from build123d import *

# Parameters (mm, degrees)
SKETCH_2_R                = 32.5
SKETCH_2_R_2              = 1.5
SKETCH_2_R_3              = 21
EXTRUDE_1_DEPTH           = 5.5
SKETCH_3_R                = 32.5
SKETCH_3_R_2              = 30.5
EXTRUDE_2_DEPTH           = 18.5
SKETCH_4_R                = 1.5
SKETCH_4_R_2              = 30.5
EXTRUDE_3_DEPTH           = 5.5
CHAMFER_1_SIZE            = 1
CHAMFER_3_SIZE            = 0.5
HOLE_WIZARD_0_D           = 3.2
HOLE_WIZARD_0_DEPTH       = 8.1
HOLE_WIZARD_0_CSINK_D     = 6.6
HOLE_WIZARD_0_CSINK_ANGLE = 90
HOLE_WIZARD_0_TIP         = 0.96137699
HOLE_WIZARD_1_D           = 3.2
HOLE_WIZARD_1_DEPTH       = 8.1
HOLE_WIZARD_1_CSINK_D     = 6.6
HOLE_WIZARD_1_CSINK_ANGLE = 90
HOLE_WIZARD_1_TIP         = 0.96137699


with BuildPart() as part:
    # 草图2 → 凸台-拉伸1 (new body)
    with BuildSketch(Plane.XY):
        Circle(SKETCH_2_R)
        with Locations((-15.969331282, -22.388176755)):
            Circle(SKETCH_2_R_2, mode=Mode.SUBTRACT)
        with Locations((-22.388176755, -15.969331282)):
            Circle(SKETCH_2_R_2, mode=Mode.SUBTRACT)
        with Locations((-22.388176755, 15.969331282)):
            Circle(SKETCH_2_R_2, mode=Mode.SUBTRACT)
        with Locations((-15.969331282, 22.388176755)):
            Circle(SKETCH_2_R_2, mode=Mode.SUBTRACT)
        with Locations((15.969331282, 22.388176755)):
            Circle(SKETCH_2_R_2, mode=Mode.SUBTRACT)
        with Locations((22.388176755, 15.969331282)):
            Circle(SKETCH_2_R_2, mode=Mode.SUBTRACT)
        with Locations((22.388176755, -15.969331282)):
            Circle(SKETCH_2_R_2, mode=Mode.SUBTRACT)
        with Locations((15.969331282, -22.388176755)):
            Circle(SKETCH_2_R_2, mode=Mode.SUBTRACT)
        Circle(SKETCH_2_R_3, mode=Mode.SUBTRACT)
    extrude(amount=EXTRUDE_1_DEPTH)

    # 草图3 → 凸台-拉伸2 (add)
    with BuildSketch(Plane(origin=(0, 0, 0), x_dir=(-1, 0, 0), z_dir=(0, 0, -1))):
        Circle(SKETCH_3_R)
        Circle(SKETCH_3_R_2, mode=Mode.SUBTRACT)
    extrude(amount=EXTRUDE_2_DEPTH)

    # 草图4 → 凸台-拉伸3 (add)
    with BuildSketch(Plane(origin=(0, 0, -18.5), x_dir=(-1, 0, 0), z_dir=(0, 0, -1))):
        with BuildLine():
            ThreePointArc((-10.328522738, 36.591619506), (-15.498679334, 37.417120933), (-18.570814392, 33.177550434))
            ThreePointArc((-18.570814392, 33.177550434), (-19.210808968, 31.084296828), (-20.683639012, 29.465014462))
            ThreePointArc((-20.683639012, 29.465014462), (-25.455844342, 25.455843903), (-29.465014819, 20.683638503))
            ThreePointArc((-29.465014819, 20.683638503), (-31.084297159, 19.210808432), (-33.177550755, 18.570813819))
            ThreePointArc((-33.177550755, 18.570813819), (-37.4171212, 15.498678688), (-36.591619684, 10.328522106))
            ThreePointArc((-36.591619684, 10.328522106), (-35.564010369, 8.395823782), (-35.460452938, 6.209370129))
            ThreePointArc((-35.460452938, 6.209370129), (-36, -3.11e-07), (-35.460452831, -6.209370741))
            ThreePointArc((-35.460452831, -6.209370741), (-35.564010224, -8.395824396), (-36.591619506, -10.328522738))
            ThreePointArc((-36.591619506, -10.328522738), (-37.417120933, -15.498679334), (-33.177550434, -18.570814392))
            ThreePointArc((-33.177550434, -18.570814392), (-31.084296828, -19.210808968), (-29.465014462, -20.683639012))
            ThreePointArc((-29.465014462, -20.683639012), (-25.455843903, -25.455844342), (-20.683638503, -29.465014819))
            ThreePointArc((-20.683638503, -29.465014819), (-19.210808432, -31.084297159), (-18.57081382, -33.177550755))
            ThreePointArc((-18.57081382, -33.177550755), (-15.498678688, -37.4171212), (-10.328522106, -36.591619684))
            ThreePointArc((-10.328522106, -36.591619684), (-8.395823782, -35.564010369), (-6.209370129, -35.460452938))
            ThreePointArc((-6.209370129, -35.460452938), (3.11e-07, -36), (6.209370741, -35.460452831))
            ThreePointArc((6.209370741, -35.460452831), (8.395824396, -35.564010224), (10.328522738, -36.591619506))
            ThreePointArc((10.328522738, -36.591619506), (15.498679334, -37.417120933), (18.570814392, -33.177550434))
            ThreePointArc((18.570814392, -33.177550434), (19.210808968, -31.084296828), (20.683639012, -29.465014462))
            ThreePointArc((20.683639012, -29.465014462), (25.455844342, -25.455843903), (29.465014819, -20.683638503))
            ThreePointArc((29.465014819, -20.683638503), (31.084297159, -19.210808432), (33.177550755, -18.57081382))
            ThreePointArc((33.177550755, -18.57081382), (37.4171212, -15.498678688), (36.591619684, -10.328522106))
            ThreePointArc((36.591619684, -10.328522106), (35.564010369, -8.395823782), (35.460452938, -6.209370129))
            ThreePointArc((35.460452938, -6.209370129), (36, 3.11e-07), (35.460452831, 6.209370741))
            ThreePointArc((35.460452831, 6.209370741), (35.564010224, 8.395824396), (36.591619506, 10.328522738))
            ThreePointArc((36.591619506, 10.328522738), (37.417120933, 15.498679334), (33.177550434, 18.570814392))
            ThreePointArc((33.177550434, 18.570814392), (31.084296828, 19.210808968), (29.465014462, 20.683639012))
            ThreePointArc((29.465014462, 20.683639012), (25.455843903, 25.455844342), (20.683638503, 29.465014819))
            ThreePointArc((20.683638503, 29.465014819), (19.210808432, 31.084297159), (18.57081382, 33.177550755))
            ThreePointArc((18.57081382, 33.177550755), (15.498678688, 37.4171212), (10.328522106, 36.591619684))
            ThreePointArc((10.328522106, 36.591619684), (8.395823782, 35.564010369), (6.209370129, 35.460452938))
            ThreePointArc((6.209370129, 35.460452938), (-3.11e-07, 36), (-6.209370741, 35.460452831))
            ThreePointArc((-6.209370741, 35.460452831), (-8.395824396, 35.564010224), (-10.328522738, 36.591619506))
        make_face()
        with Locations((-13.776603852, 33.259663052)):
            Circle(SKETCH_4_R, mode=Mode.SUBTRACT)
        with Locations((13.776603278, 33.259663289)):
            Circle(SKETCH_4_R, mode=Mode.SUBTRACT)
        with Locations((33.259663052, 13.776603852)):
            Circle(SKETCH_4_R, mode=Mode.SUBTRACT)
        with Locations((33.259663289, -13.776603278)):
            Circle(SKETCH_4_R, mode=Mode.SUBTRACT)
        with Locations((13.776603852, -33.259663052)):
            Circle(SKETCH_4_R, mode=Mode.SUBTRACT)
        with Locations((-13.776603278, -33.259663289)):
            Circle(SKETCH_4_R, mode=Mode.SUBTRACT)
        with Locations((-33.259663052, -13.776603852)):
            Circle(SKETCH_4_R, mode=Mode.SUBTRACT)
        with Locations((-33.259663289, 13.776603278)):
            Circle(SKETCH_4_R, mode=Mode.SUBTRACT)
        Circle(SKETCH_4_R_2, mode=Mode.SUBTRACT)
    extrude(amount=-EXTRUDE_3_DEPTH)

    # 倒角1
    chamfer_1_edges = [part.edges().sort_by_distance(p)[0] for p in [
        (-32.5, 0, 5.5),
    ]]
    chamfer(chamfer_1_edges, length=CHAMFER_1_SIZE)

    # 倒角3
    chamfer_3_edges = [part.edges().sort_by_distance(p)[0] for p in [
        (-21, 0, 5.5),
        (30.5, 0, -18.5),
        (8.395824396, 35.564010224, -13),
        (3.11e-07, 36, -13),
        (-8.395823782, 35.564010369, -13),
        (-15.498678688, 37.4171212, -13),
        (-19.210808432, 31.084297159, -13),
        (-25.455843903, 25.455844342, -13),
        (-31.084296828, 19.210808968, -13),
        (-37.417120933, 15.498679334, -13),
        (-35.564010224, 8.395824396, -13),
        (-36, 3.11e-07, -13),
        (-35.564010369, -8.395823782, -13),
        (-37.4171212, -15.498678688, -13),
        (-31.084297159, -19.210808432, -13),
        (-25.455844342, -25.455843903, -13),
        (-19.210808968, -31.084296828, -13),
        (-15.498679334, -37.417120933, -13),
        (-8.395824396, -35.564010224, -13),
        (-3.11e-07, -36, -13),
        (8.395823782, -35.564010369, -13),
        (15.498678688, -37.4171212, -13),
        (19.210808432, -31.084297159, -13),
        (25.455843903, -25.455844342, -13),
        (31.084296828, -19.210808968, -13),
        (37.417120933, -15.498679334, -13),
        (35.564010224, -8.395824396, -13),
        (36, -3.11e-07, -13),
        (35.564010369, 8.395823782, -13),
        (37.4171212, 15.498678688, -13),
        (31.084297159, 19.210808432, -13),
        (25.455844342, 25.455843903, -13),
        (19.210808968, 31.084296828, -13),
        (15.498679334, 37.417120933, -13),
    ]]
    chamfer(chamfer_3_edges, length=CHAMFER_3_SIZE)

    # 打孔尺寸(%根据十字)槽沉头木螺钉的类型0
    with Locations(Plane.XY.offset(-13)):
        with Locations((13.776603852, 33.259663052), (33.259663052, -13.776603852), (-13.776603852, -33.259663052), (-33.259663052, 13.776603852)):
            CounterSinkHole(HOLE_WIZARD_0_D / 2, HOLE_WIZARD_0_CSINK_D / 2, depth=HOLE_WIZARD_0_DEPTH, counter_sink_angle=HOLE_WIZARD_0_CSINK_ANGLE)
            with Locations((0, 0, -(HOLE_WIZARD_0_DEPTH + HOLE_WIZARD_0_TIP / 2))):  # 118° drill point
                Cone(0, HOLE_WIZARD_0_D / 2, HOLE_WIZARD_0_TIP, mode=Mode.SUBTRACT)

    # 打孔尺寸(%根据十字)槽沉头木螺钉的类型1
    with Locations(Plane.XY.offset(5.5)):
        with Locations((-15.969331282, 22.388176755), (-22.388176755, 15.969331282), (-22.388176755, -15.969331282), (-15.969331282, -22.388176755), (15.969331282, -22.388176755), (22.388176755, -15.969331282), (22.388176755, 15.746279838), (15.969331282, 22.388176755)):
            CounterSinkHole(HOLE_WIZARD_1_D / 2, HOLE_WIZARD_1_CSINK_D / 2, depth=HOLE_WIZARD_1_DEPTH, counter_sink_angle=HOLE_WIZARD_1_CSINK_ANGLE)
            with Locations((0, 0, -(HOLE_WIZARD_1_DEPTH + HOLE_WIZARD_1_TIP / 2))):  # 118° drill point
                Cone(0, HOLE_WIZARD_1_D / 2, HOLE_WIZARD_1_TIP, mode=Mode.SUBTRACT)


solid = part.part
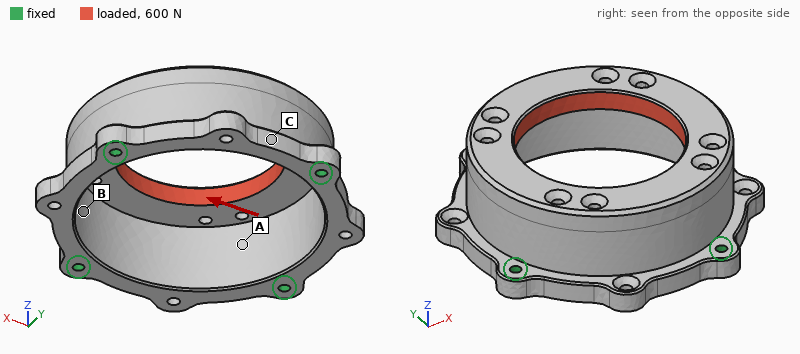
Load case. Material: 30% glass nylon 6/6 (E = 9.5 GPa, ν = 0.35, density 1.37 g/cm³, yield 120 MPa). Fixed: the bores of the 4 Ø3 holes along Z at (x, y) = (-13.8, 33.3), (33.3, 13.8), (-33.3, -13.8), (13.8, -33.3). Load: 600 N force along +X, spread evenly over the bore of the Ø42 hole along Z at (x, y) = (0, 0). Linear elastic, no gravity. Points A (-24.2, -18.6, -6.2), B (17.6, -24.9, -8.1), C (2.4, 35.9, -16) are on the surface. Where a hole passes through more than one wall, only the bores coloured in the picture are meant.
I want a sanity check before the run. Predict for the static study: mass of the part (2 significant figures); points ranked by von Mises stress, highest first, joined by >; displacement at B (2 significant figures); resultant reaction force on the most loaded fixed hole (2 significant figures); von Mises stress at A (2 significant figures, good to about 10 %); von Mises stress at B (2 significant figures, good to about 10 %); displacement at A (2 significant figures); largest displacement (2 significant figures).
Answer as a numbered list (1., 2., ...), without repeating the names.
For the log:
1. 31 g
2. A > B > C
3. 13 µm
4. 210 N
5. 5.9 MPa
6. 2.5 MPa
7. 14 µm
8. 36 µm
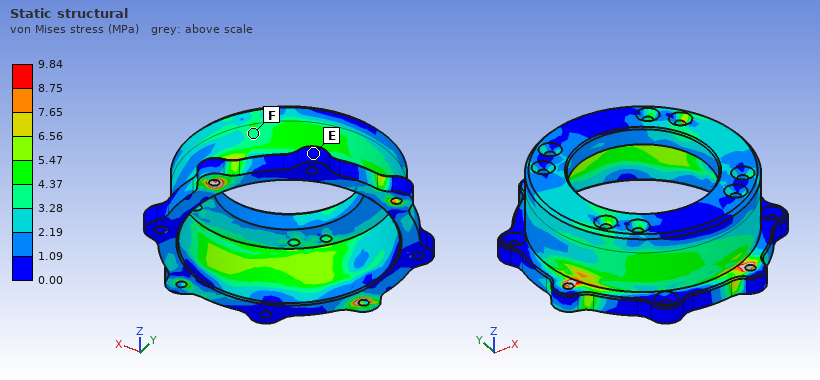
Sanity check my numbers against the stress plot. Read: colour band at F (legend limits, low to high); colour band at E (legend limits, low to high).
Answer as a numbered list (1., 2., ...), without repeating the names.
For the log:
1. 3.28 to 4.37 MPa
2. 0.00 to 1.09 MPa
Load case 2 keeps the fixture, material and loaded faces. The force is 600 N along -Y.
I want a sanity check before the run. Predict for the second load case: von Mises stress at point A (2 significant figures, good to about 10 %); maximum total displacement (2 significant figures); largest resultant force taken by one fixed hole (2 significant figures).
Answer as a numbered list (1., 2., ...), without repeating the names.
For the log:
1. 2.3 MPa
2. 36 µm
3. 210 N
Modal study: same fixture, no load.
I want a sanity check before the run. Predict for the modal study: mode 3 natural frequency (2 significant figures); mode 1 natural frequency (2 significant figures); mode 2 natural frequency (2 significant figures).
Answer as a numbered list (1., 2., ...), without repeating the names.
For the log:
1. 5200 Hz
2. 4900 Hz
3. 5200 Hz
